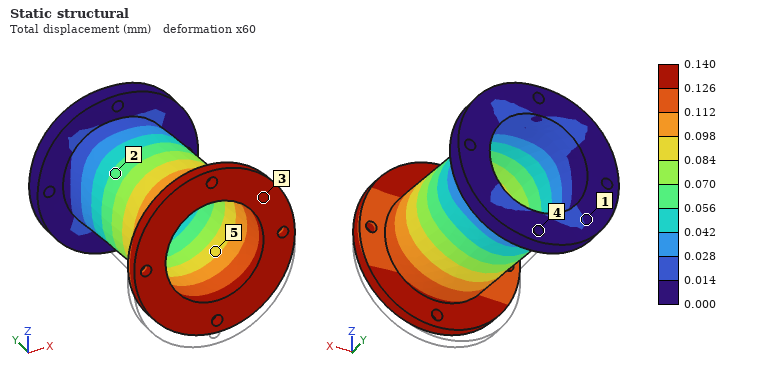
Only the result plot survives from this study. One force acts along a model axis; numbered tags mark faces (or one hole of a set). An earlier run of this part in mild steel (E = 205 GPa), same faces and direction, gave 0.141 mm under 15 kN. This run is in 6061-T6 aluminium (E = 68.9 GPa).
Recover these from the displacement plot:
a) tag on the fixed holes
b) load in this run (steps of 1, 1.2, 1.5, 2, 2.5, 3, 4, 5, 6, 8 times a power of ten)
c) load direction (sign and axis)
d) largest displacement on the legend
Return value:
4
5 kN
+Z
0.140 mm
